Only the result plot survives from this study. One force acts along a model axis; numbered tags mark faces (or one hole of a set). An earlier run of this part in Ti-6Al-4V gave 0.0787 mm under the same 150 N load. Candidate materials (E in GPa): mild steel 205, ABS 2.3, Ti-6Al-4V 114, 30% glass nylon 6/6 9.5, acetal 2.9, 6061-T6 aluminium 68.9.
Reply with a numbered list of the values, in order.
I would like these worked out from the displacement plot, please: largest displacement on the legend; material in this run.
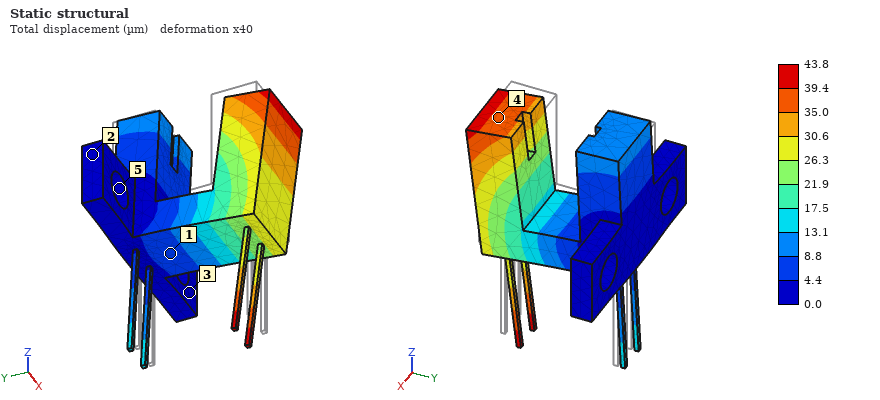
1. 43.8 µm
2. mild steel
